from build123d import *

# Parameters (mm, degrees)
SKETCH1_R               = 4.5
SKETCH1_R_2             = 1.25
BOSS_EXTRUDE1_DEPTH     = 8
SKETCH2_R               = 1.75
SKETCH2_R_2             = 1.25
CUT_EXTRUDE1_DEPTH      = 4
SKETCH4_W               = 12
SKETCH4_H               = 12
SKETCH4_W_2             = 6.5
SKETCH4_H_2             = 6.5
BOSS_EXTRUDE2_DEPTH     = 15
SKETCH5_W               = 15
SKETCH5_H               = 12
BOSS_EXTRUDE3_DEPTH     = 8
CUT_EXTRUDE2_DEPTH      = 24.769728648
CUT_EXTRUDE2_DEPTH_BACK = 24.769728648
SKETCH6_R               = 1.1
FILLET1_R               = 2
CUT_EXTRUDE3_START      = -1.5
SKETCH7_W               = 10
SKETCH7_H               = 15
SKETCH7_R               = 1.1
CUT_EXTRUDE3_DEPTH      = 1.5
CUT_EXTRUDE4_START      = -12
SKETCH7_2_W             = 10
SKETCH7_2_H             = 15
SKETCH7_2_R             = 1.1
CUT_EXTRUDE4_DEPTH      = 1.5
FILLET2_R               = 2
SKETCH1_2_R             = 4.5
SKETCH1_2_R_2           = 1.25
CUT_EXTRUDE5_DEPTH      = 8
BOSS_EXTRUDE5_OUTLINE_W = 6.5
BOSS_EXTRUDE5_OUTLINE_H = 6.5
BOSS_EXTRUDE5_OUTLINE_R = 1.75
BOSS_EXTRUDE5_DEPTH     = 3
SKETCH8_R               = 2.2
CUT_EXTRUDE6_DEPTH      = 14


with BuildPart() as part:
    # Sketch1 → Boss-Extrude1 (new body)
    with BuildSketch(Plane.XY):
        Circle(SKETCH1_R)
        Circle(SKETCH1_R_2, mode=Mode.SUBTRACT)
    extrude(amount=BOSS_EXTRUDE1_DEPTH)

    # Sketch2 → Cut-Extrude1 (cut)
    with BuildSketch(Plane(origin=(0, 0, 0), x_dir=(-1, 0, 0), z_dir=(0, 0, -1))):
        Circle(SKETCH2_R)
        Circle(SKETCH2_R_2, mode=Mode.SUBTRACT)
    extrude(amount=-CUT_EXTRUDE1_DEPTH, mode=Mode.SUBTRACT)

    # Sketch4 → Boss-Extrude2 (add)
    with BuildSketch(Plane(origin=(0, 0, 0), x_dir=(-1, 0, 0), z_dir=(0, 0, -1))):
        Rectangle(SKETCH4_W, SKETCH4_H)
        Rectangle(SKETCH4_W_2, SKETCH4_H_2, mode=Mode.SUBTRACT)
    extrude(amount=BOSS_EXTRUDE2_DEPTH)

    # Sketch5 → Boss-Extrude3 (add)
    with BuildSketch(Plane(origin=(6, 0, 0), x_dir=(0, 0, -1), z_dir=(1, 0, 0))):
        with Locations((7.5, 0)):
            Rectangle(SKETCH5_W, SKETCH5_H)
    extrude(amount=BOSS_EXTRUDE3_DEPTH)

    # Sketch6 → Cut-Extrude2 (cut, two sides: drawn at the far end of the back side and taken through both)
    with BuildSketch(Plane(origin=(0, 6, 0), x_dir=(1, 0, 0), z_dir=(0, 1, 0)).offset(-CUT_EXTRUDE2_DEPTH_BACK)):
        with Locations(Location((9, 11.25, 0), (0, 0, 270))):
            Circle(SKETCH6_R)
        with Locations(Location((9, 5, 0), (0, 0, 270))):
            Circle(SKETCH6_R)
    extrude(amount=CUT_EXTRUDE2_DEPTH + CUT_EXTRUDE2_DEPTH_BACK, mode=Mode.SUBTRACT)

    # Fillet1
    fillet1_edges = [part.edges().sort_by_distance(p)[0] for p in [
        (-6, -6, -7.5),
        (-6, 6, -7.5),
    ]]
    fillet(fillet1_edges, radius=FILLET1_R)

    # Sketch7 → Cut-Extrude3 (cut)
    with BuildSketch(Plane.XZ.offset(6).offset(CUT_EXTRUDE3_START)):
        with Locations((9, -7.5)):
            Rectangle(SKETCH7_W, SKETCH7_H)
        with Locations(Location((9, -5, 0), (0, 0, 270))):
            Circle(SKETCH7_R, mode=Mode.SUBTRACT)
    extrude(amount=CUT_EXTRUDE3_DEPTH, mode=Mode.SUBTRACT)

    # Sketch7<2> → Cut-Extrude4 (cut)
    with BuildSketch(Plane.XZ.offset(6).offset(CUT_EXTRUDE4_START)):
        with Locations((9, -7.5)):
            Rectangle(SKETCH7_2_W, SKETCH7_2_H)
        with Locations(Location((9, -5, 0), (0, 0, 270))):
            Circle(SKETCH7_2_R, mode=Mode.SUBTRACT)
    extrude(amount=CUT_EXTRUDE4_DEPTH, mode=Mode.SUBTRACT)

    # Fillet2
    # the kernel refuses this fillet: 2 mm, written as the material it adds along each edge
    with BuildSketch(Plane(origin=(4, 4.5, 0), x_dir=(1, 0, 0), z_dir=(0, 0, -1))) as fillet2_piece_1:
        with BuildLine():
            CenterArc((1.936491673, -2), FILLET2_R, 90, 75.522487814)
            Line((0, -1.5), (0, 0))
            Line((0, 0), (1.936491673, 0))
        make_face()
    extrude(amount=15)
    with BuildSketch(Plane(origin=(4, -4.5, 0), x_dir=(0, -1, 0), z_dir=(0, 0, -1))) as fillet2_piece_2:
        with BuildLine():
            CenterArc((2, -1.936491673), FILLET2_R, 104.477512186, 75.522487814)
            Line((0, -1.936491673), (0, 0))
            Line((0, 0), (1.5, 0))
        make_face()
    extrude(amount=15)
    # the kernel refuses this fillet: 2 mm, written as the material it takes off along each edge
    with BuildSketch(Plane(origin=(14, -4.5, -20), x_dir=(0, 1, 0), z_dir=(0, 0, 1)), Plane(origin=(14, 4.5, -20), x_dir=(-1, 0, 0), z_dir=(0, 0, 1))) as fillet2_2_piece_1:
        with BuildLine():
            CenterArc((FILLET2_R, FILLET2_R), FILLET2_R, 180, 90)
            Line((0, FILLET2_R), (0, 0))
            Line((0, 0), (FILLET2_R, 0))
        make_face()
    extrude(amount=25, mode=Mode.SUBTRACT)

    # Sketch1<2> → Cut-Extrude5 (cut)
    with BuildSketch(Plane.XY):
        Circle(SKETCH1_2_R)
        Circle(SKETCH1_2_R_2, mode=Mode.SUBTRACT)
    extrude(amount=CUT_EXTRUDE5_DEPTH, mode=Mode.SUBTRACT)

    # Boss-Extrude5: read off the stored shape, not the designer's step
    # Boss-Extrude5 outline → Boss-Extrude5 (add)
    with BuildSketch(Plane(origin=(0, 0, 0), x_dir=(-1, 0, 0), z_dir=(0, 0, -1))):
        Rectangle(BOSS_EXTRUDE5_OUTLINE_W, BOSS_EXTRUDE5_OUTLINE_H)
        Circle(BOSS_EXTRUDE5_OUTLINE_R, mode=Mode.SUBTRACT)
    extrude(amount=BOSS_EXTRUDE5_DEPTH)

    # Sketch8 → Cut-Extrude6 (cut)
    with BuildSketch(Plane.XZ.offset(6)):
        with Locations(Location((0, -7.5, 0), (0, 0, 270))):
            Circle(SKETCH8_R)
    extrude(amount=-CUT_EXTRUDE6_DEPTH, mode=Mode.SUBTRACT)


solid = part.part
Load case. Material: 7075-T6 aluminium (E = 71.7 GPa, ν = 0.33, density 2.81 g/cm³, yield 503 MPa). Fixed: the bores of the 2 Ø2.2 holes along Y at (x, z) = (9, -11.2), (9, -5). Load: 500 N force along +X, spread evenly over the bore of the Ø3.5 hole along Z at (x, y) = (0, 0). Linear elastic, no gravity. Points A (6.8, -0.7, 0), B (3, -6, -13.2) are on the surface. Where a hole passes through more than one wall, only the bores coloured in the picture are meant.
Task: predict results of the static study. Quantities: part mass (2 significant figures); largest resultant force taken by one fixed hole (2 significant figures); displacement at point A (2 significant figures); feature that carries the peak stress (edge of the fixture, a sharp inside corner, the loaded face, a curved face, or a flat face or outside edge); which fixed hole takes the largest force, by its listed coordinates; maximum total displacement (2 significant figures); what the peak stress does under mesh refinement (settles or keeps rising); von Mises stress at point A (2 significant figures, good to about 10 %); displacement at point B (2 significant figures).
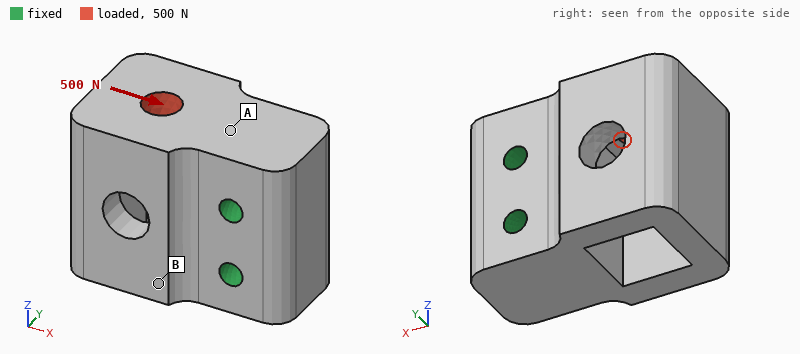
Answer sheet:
6.8 g
670 N
1.5 µm
edge of the fixture
(9, -5)
4.5 µm
keeps rising
9.3 MPa
0.76 µm
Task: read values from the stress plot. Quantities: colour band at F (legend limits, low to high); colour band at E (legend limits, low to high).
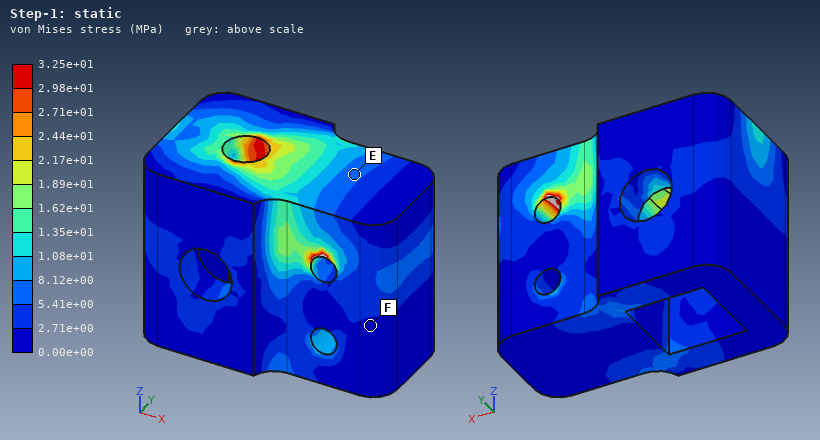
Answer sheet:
0.00e+00 to 2.71e+00 MPa
5.41e+00 to 8.12e+00 MPa
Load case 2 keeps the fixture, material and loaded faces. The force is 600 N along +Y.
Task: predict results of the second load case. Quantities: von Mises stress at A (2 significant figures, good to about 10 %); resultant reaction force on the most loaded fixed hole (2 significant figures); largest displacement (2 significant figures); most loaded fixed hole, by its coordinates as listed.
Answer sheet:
19 MPa
570 N
14 µm
(9, -5)
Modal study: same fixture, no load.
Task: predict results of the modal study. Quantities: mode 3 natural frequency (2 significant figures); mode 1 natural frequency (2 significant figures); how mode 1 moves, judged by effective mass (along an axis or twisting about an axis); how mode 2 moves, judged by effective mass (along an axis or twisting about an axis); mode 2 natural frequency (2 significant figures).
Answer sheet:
35 kHz
18 kHz
along Y
along Z
24 kHz
